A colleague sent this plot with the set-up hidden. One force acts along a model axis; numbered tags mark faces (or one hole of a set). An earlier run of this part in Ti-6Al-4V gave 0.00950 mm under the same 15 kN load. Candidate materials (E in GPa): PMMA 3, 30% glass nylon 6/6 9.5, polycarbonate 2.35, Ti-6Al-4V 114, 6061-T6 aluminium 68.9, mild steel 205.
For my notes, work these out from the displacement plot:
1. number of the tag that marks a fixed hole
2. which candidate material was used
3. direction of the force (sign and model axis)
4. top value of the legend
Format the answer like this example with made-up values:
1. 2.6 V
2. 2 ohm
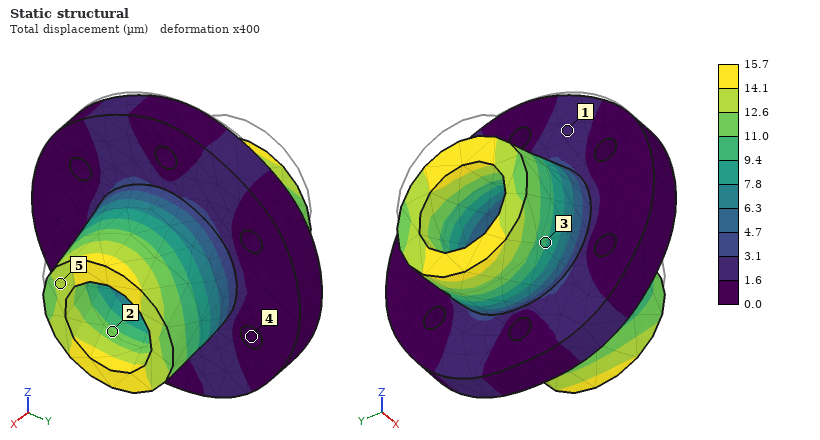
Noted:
1. 4
2. 6061-T6 aluminium
3. -Z
4. 15.7 µm
